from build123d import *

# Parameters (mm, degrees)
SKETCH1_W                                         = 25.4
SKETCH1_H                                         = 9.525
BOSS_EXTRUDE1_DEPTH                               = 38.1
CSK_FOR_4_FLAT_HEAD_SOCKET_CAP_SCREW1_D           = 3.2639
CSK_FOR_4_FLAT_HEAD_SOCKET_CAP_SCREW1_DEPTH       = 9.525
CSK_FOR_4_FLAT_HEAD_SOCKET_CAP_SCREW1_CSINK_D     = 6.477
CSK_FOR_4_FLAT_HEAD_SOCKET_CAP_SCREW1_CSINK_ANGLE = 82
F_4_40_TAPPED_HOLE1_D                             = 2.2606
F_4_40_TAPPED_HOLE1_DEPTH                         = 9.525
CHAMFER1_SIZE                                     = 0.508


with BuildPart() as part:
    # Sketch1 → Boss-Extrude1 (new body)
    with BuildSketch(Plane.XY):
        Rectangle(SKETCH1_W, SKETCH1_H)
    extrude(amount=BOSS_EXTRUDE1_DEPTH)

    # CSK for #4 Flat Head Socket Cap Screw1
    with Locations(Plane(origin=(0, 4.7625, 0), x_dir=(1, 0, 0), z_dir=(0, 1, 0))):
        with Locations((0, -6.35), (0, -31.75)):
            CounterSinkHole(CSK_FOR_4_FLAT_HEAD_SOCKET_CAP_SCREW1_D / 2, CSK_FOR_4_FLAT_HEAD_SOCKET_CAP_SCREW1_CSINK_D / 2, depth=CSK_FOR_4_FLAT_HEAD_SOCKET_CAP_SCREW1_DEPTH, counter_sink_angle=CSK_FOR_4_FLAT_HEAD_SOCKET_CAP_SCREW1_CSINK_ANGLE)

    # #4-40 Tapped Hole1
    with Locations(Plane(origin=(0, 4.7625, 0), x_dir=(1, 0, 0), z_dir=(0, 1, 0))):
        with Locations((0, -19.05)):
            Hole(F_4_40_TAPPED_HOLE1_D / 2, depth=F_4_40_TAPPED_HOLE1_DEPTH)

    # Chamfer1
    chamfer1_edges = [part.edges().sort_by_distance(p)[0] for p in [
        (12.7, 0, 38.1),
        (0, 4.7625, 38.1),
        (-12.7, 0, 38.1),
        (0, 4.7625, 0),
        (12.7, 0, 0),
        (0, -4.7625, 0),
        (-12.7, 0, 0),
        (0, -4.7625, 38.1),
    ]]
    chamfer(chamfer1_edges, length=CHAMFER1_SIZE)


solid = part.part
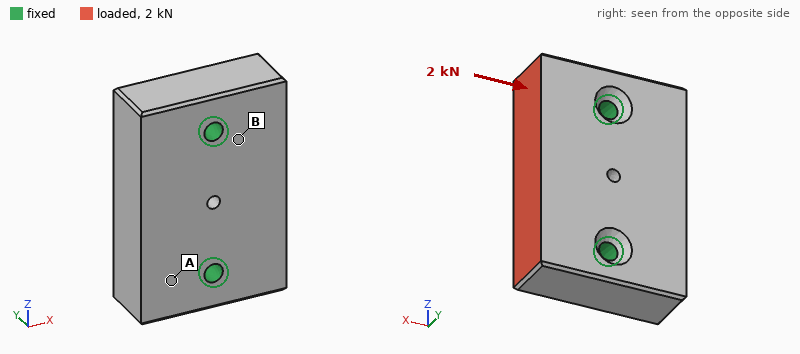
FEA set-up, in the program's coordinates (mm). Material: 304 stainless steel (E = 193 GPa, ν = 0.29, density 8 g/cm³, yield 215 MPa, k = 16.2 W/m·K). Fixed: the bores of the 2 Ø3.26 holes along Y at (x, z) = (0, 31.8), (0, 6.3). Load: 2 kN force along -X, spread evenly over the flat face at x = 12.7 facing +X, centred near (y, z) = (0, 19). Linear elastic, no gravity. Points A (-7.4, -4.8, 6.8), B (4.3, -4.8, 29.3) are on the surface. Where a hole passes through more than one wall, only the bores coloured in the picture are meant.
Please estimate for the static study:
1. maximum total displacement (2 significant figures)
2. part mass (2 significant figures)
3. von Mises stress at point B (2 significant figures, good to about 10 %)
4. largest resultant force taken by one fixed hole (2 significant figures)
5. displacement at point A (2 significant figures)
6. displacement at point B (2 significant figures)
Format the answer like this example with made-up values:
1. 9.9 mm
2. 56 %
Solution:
1. 0.84 µm
2. 72 g
3. 8.3 MPa
4. 1.0 kN
5. 0.13 µm
6. 0.19 µm
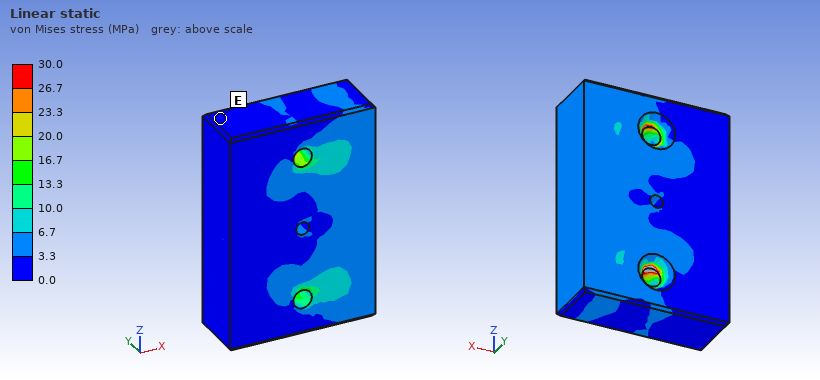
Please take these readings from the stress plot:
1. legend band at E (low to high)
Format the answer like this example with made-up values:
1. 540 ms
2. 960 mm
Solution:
1. 0.0 to 3.3 MPa
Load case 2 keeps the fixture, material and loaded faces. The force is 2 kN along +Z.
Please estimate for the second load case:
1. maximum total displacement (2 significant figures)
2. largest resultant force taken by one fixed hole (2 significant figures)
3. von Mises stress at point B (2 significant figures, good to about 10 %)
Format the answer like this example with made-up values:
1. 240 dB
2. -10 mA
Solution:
1. 2.1 µm
2. 1.4 kN
3. 15 MPa
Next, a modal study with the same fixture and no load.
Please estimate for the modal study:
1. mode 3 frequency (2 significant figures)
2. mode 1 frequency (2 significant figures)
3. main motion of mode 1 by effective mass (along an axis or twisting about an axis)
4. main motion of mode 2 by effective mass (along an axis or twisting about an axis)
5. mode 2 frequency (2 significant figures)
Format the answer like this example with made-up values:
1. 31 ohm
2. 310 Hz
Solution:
1. 34 kHz
2. 20 kHz
3. twisting about Z
4. along Y
5. 27 kHz
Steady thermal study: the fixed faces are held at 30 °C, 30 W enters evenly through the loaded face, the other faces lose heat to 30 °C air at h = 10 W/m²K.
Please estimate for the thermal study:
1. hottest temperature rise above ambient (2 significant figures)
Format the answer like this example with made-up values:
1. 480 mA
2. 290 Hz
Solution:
1. 83 K
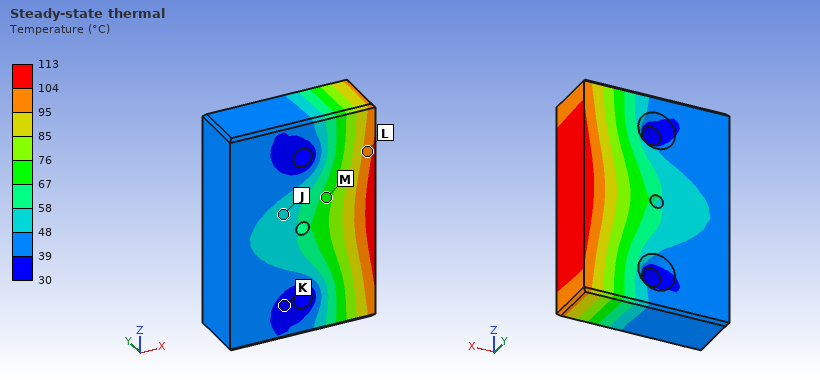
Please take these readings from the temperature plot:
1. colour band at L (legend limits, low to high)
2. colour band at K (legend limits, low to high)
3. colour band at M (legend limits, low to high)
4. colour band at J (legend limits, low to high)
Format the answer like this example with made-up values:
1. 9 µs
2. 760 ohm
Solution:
1. 95 to 104 °C
2. 30 to 39 °C
3. 67 to 76 °C
4. 48 to 58 °C
